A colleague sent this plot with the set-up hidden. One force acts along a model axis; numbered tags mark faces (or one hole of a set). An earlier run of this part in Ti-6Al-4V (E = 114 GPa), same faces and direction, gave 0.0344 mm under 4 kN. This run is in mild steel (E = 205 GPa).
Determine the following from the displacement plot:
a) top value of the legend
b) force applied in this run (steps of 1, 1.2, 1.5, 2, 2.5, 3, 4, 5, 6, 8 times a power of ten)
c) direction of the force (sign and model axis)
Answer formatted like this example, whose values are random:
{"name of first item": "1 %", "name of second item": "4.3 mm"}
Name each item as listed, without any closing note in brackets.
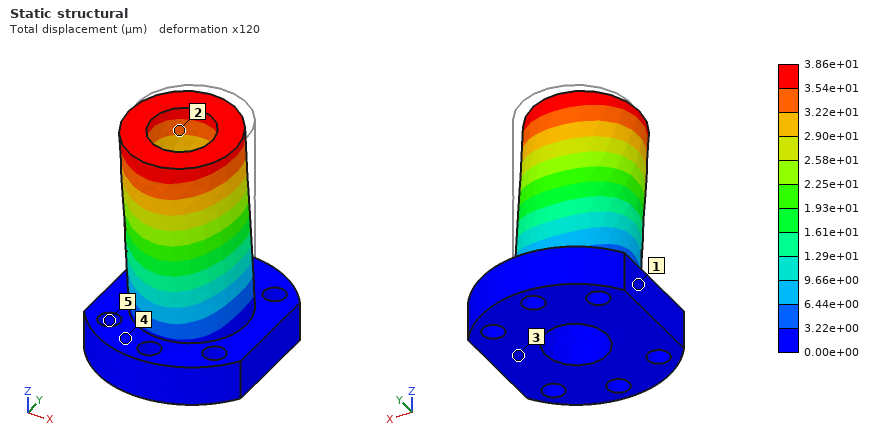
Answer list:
{"top value of the legend": "3.86e+01 µm", "force applied in this run": "8 kN", "direction of the force": "-Y"}
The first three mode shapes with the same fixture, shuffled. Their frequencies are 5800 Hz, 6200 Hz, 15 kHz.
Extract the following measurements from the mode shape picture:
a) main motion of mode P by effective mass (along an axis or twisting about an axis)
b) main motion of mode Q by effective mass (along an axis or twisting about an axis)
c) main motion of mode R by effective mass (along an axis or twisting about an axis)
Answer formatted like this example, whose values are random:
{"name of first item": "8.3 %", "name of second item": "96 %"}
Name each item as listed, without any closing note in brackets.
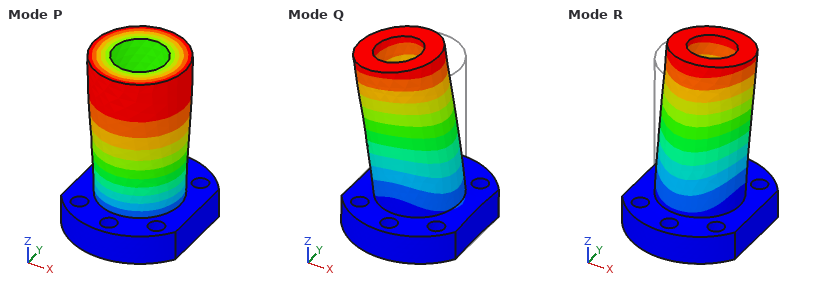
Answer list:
{"main motion of mode P by effective mass": "twisting about Z", "main motion of mode Q by effective mass": "along X", "main motion of mode R by effective mass": "along Y"}
